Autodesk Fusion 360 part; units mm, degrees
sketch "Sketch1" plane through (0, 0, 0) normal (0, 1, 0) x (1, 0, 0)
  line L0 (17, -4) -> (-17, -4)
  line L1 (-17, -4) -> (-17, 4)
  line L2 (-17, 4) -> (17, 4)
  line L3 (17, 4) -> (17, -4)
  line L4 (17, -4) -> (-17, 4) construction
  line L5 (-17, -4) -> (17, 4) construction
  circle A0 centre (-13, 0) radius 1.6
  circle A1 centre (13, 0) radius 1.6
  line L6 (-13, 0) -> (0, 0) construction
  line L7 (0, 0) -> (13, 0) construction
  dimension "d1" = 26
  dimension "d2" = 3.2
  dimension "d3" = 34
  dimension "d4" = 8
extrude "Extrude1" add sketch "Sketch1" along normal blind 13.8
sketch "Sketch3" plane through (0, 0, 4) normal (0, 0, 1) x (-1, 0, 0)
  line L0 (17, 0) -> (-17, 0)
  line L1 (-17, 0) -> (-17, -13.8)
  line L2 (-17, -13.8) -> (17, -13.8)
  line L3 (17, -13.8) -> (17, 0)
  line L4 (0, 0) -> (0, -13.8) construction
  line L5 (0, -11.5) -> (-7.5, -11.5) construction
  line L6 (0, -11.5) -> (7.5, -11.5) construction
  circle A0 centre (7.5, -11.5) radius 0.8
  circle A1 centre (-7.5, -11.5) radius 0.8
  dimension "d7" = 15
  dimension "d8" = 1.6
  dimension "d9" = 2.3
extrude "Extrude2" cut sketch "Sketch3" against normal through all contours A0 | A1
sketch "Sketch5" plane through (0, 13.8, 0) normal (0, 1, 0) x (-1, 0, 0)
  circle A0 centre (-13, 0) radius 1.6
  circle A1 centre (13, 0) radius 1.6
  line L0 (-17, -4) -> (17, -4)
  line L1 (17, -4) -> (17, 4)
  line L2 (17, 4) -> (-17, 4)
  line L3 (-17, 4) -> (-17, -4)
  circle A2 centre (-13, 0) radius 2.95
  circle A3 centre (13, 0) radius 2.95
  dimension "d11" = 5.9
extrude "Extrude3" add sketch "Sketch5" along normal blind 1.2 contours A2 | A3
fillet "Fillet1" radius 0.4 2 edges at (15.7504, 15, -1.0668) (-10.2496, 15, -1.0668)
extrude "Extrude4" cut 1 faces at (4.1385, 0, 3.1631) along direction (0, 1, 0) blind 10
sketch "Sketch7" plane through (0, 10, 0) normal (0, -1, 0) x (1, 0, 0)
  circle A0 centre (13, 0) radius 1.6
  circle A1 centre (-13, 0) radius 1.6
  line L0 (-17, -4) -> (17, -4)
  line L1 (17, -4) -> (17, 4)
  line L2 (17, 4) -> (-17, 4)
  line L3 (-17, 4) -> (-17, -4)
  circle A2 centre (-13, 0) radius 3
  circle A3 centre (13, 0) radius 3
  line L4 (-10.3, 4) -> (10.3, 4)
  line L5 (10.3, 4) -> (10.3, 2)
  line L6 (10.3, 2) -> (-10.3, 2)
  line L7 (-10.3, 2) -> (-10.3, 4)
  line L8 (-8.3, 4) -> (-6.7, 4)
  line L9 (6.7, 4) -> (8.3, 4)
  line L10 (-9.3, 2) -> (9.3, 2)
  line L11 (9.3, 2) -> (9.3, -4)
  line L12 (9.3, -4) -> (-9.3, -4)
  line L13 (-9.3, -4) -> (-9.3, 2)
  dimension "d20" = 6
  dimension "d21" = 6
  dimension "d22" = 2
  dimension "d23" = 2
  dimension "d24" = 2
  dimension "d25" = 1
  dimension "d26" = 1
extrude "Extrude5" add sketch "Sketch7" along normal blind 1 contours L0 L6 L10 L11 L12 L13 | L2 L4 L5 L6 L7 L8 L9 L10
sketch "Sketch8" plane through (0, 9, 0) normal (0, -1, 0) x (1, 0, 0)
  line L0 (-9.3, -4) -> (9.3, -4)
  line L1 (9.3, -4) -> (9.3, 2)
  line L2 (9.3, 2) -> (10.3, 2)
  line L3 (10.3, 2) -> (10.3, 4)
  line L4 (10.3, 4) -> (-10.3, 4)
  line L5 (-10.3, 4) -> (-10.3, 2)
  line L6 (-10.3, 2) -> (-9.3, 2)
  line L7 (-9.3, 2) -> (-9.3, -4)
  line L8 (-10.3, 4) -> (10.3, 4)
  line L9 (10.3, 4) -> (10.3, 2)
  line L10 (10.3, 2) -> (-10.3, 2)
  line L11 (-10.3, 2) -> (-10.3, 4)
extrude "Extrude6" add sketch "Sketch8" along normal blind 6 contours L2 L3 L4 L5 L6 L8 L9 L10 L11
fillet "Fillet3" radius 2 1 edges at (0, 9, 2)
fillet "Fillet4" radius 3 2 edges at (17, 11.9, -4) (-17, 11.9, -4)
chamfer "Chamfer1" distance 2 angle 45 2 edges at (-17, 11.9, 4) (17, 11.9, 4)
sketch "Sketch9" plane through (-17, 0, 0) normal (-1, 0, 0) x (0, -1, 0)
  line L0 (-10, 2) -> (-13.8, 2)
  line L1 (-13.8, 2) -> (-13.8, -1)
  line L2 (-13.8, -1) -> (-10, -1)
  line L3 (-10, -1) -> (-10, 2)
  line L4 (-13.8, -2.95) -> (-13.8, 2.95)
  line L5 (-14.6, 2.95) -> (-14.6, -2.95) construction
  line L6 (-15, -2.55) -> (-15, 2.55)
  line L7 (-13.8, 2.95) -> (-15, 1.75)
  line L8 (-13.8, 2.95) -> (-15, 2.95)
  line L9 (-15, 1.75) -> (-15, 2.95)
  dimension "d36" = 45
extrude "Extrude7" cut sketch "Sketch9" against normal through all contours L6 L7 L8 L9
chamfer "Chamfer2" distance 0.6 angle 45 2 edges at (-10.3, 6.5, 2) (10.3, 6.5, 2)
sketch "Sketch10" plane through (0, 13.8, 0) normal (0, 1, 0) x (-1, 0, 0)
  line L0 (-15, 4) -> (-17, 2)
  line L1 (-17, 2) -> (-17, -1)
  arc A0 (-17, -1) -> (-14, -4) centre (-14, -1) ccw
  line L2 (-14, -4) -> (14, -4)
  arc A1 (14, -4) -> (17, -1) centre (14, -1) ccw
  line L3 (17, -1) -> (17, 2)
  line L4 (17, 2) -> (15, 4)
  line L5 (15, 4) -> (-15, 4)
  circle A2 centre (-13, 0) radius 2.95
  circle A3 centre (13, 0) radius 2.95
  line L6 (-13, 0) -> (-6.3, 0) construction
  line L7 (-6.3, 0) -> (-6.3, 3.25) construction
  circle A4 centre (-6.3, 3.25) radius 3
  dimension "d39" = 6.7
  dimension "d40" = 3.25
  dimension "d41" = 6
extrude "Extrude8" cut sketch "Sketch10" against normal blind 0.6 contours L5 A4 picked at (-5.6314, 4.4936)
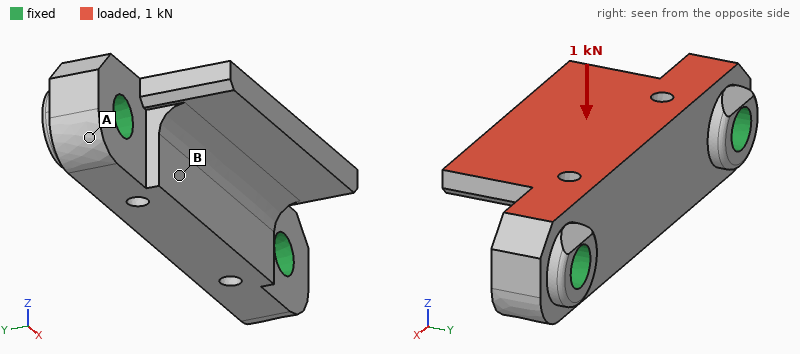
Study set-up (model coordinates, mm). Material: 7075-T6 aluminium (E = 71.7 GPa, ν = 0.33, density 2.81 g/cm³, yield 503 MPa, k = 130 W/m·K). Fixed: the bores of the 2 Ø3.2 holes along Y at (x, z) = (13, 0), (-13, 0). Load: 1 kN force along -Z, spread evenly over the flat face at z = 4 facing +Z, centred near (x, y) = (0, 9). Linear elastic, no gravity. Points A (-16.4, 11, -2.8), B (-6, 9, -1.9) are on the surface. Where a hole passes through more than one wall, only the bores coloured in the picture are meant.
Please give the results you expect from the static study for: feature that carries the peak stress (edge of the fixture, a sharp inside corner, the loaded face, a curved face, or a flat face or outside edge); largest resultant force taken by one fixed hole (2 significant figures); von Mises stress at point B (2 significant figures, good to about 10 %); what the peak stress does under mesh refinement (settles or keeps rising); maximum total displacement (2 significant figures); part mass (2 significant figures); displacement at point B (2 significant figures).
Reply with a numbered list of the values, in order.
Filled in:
1. edge of the fixture
2. 500 N
3. 40 MPa
4. keeps rising
5. 46 µm
6. 3.8 g
7. 12 µm
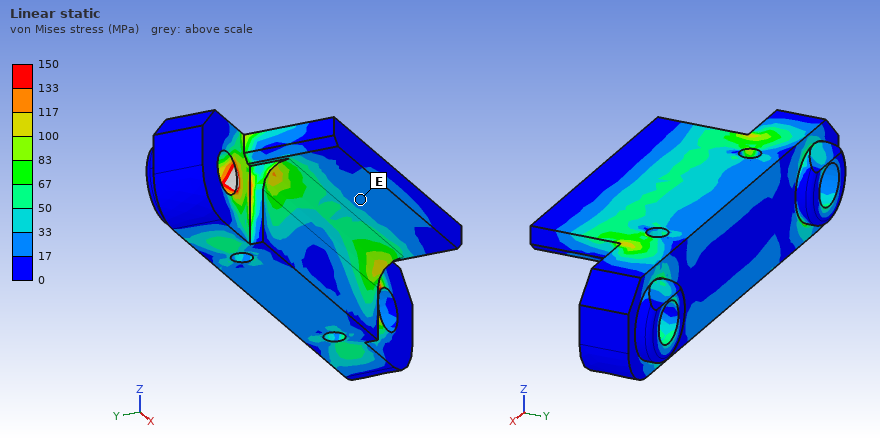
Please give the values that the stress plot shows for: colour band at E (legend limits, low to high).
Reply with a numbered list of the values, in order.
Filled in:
1. 17 to 33 MPa
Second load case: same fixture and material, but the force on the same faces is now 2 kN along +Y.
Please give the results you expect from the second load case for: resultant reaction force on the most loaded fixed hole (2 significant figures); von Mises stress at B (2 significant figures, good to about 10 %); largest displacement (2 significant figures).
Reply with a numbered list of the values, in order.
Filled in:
1. 1.1 kN
2. 51 MPa
3. 66 µm
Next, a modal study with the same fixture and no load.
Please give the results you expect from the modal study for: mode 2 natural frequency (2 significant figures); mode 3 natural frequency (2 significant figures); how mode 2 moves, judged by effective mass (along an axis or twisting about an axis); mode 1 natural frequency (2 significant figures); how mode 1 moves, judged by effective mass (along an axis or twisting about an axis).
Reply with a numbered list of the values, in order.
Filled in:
1. 34 kHz
2. 40 kHz
3. along Y
4. 23 kHz
5. along Z
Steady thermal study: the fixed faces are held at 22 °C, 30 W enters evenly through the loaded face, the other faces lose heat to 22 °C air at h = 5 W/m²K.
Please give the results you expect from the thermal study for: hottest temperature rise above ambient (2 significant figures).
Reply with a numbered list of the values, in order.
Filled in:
1. 32 K
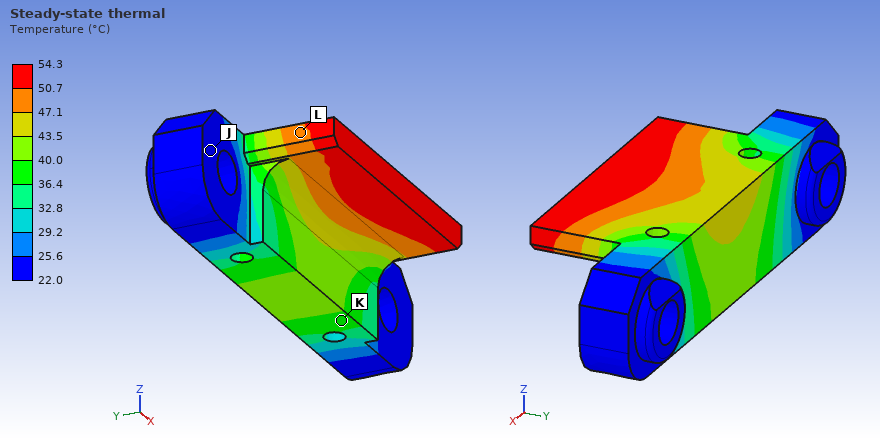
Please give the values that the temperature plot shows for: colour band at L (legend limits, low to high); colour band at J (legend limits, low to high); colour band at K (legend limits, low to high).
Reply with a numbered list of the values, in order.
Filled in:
1. 47.1 to 50.7 °C
2. 22.0 to 25.6 °C
3. 36.4 to 40.0 °C
